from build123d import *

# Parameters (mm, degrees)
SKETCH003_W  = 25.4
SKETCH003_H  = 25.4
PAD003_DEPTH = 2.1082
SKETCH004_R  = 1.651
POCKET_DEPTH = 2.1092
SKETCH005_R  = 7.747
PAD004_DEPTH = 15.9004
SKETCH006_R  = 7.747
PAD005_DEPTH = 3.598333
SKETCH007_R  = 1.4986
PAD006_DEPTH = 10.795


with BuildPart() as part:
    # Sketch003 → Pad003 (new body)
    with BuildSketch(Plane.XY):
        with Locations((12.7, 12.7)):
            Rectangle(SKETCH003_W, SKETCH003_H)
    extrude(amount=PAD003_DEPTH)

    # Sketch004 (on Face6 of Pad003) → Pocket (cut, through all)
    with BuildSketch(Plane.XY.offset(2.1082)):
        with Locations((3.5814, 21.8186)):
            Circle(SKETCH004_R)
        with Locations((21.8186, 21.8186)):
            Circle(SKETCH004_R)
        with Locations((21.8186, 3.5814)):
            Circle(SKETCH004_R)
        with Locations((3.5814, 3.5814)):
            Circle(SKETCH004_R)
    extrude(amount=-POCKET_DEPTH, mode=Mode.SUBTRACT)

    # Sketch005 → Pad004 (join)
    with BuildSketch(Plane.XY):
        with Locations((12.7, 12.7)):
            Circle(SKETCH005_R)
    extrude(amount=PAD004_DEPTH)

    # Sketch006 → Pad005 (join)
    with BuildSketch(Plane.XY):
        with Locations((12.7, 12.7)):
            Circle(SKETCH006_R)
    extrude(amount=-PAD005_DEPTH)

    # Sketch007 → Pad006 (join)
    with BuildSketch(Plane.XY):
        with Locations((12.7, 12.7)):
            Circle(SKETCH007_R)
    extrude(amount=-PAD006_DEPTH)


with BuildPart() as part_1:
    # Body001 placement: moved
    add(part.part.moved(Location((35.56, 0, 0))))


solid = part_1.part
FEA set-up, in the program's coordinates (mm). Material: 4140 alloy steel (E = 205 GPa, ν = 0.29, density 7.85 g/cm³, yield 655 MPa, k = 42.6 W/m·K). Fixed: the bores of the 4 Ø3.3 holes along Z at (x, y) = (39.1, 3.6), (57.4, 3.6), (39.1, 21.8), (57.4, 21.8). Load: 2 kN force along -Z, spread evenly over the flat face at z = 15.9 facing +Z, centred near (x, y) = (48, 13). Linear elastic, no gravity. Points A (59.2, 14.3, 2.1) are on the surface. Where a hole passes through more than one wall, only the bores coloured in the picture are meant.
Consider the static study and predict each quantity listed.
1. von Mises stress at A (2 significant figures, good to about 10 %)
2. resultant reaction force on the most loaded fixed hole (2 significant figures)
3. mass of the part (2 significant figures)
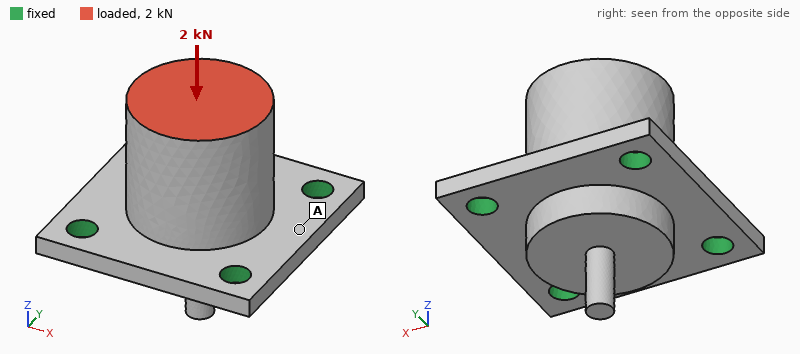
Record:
37 MPa
500 N
36 g
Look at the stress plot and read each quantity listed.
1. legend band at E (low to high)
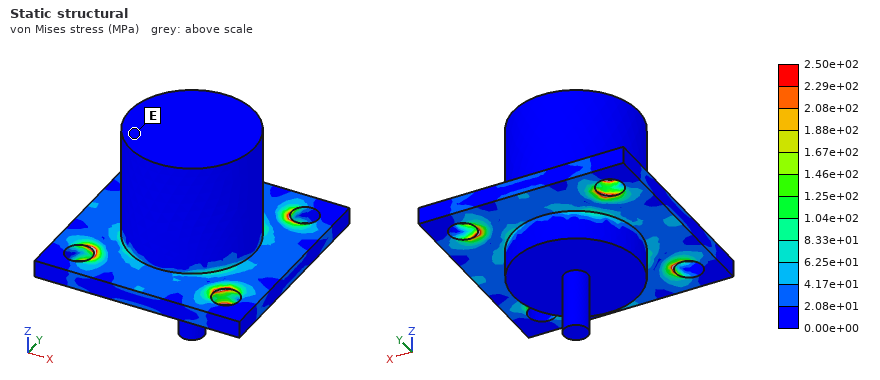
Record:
0.00e+00 to 2.08e+01 MPa
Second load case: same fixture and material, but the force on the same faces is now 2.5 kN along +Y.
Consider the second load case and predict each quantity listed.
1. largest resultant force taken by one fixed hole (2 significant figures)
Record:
1.4 kN
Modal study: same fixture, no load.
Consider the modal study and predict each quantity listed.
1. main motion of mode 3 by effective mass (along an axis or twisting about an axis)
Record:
along Z
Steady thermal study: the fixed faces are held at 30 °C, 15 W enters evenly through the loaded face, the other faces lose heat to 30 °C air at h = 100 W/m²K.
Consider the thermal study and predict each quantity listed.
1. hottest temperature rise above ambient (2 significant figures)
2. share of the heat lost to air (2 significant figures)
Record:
43 K
23 %
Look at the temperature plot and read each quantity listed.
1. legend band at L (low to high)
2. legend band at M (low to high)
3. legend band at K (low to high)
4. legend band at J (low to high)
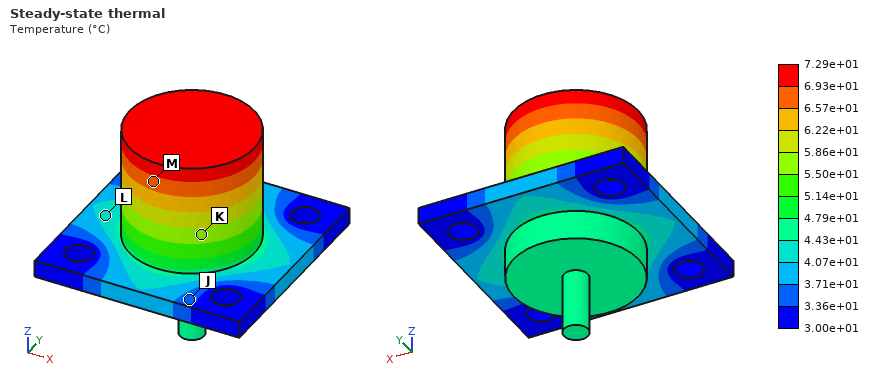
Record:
4.07e+01 to 4.43e+01 °C
6.57e+01 to 6.93e+01 °C
5.50e+01 to 5.86e+01 °C
3.36e+01 to 3.71e+01 °C
